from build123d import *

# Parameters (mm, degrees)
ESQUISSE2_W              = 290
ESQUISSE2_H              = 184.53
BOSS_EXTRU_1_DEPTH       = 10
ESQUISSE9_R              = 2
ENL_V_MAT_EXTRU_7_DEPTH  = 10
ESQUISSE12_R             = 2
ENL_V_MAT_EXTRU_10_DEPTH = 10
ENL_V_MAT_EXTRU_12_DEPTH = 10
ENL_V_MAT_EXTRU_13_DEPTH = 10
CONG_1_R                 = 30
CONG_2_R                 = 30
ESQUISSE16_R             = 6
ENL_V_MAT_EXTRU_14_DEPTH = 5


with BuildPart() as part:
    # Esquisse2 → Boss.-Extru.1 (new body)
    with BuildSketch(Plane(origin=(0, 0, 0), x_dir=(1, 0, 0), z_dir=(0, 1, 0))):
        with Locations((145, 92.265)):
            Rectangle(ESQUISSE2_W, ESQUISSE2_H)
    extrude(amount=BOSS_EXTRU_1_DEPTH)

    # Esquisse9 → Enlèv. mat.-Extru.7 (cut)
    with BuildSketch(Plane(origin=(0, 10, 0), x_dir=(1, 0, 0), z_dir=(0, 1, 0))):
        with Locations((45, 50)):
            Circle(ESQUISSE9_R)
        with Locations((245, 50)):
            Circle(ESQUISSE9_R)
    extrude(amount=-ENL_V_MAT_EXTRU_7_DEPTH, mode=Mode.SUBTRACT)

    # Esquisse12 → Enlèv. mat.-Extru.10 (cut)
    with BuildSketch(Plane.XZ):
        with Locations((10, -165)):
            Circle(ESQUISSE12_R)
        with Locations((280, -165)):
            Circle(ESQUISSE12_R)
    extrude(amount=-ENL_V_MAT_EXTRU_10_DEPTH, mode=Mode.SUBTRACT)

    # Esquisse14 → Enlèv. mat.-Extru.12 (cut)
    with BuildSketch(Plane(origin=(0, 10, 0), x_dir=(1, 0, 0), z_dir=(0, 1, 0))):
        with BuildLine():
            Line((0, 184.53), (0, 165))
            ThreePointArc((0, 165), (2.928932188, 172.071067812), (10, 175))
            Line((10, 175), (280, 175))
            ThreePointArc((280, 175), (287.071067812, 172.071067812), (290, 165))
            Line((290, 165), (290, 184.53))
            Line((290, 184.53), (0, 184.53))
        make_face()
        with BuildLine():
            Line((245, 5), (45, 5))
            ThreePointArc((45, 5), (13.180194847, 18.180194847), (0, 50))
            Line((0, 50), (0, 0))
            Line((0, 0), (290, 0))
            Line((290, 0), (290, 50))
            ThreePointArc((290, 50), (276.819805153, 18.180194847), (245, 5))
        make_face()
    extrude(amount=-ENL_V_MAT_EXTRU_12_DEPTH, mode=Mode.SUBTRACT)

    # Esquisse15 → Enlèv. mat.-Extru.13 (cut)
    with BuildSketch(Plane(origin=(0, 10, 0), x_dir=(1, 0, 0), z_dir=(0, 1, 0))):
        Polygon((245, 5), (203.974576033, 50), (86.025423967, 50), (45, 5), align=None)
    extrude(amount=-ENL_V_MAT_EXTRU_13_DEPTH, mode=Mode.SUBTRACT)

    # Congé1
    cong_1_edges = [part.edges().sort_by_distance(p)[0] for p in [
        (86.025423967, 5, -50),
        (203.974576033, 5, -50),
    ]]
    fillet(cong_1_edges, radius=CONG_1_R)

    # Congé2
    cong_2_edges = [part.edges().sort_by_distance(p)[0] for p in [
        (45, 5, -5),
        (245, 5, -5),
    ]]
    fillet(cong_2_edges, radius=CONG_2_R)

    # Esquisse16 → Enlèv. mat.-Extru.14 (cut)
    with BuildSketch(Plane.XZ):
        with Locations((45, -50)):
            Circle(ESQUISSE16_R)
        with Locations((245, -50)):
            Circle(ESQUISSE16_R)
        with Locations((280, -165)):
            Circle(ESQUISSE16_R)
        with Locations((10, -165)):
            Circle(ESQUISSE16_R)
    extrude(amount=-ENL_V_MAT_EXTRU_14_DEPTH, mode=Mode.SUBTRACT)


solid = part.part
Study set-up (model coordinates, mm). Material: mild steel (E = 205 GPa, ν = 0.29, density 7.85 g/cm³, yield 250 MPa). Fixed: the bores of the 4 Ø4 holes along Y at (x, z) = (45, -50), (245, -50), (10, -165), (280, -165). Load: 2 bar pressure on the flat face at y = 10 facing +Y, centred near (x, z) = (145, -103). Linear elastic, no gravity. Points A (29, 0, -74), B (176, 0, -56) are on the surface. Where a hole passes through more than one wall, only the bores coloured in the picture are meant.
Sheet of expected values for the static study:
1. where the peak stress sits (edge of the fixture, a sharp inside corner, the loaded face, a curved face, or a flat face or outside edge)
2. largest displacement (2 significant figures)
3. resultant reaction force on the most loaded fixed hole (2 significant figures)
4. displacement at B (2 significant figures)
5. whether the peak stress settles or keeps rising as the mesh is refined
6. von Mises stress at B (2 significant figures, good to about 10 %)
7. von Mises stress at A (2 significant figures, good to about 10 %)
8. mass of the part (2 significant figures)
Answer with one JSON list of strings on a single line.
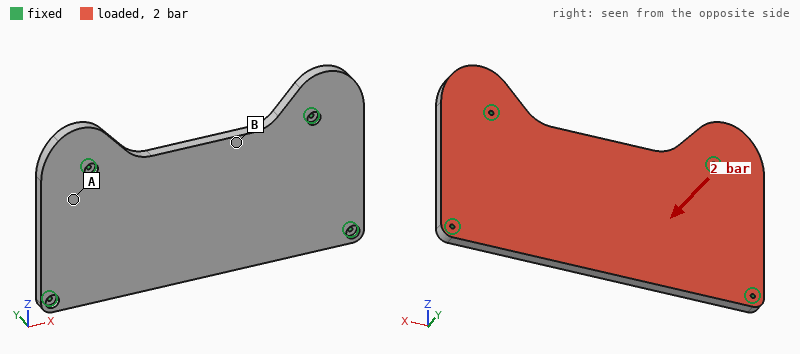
["edge of the fixture", "0.30 mm", "4.2 kN", "0.13 mm", "keeps rising", "42 MPa", "19 MPa", "3.2 kg"]
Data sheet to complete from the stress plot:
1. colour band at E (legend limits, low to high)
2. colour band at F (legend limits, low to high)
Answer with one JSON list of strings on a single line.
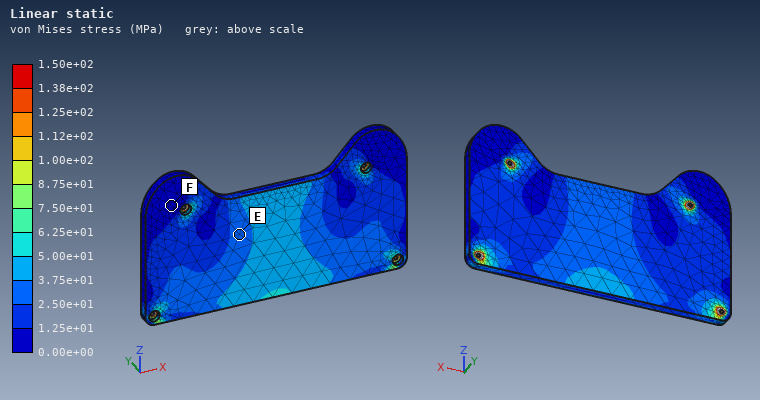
["2.50e+01 to 3.75e+01 MPa", "0.00e+00 to 1.25e+01 MPa"]
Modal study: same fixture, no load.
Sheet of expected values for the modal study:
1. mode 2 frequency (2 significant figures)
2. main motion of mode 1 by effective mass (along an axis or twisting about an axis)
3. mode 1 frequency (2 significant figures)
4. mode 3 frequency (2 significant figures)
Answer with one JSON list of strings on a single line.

["1400 Hz", "along Y", "580 Hz", "1600 Hz"]
